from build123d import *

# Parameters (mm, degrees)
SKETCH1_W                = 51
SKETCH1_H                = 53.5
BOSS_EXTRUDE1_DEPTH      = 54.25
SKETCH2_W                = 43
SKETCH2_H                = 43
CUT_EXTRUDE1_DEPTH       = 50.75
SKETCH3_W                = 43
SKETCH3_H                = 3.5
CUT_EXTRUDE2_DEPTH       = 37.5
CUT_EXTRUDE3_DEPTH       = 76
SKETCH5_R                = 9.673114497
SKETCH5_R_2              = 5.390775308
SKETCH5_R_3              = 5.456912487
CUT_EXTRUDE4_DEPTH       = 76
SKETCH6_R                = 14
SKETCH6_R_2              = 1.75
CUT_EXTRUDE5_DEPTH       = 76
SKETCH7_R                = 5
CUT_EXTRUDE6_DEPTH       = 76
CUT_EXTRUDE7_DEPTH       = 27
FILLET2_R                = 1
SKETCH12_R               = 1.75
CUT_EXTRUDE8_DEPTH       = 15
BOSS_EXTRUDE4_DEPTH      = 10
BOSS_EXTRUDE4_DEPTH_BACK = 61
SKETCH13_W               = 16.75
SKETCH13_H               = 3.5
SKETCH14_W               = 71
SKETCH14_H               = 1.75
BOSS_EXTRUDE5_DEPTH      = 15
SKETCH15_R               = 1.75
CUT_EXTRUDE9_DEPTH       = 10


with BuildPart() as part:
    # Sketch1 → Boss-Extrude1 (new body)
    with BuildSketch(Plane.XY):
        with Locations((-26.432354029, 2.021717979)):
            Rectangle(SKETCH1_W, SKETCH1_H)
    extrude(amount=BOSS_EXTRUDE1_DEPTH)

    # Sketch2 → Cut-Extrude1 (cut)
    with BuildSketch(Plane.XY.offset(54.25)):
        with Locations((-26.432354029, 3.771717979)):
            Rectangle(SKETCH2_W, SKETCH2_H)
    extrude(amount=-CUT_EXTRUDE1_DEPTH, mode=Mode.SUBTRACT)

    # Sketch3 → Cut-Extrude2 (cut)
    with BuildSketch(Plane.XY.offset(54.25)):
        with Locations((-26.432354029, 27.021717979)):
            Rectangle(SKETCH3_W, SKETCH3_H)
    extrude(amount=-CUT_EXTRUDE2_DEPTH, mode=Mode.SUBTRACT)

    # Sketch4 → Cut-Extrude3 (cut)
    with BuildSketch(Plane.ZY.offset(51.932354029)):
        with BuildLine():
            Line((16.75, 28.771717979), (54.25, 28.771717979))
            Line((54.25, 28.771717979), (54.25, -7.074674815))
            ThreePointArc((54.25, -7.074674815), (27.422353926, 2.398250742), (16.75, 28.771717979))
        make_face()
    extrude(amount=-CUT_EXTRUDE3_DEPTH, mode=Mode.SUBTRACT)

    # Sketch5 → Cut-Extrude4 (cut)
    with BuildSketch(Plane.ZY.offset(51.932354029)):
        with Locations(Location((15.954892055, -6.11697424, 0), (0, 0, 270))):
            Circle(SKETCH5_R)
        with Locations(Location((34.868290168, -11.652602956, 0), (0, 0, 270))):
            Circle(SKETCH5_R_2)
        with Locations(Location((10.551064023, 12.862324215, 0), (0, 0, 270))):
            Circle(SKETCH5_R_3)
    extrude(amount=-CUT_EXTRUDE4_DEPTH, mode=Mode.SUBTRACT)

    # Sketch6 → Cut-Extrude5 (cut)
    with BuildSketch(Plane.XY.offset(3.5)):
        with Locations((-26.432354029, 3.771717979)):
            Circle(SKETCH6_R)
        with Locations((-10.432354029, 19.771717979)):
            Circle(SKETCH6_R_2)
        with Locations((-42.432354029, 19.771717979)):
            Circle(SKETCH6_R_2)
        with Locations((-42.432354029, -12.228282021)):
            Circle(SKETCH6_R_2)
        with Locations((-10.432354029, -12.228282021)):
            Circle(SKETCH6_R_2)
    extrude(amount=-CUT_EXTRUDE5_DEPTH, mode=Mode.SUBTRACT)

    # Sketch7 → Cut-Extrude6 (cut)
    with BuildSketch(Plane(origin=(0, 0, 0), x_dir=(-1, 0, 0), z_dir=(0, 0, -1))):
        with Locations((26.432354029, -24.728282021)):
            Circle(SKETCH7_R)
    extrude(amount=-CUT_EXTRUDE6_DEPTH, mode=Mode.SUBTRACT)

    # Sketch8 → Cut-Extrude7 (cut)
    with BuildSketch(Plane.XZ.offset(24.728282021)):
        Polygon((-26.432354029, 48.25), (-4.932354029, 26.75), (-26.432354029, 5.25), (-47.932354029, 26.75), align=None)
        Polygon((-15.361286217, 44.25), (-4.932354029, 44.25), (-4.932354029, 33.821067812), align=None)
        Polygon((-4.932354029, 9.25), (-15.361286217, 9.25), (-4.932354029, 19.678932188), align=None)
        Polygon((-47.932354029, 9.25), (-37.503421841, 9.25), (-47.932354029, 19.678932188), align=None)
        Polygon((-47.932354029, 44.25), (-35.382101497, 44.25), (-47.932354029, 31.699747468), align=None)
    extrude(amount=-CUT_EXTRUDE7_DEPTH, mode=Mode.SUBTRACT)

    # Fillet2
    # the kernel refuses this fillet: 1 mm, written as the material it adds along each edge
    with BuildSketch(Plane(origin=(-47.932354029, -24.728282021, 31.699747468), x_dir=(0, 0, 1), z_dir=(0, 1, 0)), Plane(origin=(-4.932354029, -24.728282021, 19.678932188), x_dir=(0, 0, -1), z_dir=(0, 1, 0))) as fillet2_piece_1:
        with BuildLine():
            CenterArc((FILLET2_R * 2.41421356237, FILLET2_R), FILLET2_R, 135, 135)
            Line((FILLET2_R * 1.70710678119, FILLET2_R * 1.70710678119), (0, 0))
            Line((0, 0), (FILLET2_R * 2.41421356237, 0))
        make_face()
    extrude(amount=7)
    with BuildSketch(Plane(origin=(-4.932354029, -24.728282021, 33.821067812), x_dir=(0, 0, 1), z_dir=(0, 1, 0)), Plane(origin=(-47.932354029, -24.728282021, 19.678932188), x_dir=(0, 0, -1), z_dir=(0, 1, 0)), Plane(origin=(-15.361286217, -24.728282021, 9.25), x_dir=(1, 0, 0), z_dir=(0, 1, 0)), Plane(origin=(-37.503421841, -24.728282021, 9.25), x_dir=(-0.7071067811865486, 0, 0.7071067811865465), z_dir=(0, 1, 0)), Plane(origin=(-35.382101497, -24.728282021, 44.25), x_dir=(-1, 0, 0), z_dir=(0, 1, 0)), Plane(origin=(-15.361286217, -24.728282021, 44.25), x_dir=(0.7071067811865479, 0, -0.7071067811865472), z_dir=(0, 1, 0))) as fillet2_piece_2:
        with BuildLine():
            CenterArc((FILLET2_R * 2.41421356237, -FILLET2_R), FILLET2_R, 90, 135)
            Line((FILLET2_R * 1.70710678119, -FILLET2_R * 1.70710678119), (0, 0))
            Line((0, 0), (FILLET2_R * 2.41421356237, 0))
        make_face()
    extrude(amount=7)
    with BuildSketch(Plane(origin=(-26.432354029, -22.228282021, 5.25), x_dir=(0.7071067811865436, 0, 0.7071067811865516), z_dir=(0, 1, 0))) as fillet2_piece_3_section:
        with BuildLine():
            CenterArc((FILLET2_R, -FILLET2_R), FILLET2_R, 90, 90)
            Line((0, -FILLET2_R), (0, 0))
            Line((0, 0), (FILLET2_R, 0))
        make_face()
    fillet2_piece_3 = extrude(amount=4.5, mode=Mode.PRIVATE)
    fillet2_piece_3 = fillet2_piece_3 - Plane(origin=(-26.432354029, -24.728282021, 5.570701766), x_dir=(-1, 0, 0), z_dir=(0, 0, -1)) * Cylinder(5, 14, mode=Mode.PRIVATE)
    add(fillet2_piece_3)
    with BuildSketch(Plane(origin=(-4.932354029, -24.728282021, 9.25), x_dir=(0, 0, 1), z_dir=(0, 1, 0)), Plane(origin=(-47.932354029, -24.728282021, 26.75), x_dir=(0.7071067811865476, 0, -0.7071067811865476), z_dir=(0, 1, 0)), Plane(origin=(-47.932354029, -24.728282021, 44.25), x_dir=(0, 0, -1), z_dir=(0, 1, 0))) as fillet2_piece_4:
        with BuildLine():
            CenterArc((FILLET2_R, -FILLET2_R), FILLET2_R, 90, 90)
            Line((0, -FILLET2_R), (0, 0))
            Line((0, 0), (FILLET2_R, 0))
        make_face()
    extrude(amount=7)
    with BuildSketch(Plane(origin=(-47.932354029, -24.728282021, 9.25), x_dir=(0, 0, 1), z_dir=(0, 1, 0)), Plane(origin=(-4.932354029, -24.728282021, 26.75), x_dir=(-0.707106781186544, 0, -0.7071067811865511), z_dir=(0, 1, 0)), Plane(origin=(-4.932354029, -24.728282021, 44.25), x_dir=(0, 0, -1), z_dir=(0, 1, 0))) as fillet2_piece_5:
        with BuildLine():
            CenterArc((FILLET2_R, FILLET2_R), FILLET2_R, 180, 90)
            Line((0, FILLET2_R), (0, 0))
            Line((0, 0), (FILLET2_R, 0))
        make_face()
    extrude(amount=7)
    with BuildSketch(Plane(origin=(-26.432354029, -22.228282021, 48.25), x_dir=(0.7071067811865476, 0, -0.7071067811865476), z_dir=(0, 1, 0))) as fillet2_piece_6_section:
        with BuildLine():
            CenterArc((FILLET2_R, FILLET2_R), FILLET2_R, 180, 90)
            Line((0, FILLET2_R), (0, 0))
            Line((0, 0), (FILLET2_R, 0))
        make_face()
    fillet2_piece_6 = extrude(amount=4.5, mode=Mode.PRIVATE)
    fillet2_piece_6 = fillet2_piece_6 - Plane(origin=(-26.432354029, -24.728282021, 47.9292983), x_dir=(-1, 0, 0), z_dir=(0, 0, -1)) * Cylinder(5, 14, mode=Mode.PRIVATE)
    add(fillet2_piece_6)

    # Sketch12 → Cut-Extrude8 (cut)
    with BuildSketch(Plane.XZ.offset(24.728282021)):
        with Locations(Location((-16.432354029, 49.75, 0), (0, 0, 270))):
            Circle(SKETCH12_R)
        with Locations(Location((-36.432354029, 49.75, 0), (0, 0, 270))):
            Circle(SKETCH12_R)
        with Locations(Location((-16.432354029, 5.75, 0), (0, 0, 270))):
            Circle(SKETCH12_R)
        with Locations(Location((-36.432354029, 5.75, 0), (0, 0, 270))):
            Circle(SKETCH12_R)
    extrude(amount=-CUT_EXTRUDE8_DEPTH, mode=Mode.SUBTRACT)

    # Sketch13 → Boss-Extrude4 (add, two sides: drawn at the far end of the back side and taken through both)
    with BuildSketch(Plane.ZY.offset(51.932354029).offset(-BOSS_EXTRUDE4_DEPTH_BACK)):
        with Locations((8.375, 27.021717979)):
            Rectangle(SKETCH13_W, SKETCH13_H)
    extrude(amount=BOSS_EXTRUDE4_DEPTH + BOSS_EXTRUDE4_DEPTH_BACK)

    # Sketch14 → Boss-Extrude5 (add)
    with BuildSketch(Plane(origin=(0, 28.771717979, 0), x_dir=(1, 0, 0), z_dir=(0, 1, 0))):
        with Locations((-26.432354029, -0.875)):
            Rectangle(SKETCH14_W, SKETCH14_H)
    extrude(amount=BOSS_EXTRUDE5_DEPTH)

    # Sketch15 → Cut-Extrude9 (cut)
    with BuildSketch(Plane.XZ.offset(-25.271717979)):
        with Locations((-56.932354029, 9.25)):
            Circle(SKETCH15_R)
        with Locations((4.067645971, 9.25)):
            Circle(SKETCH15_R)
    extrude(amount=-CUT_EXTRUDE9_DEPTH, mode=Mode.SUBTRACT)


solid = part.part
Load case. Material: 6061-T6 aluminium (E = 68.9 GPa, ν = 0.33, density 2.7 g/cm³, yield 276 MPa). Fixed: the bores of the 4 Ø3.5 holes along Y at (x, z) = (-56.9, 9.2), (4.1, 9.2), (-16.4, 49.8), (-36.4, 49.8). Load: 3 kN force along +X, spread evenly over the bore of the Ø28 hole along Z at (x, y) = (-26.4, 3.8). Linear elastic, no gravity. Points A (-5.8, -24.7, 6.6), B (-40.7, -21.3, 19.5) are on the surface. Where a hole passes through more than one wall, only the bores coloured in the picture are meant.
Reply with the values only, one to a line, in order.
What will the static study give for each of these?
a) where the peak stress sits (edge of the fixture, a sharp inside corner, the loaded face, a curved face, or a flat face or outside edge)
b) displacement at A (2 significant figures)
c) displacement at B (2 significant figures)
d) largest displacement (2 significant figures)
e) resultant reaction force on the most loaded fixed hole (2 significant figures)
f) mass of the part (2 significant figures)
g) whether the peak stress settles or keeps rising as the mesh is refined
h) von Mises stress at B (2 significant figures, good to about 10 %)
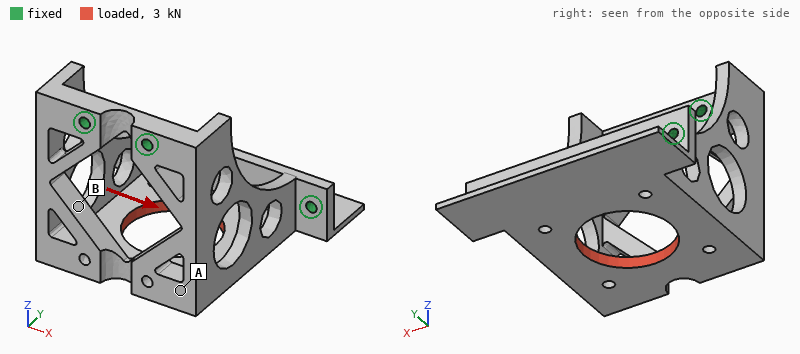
edge of the fixture
56 µm
40 µm
64 µm
1.5 kN
75 g
keeps rising
16 MPa
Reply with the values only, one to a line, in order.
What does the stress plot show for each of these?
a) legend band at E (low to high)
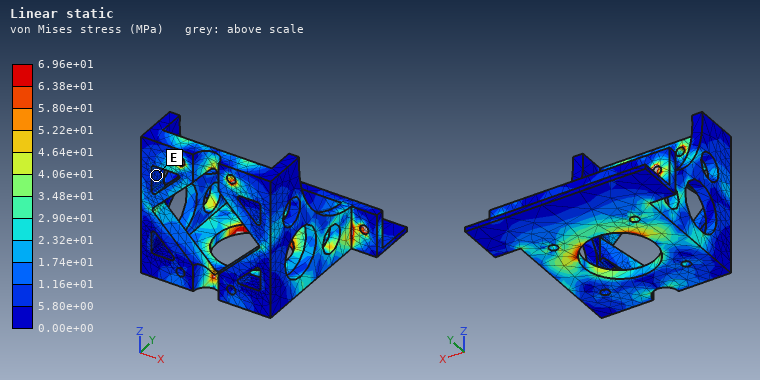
5.80e+00 to 1.16e+01 MPa
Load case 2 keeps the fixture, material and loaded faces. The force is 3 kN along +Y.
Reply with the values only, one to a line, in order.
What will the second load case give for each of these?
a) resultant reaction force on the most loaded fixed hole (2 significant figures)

1.4 kN
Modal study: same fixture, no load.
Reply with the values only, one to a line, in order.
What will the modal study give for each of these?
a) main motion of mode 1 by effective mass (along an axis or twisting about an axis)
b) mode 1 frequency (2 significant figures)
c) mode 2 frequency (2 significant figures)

along Z
5000 Hz
5400 Hz
